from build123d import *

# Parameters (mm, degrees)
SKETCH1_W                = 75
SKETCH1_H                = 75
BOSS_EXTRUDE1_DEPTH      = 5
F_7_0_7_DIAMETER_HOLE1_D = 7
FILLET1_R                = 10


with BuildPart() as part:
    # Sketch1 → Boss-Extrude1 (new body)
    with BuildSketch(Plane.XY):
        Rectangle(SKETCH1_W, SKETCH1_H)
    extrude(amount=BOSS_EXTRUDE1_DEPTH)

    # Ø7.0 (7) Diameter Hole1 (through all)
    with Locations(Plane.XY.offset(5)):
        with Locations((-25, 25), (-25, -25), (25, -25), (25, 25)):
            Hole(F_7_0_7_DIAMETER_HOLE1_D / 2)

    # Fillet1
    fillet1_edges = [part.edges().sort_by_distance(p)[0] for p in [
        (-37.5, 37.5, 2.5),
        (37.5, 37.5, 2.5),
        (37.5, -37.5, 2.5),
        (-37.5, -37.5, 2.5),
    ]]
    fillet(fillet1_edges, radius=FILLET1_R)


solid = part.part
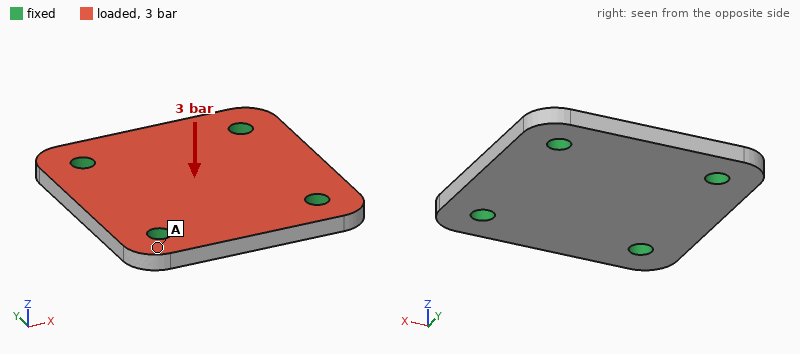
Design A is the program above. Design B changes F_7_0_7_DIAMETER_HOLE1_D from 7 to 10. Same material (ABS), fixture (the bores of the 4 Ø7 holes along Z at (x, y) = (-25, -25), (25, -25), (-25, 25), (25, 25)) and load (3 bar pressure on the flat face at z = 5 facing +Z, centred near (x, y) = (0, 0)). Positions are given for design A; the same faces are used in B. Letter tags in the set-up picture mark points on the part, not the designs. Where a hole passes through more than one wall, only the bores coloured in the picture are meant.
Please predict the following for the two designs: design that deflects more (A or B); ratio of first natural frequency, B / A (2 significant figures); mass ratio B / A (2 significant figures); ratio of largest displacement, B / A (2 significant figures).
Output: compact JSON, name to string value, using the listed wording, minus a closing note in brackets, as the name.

{"design that deflects more": "A", "ratio of first natural frequency, B / A": "1.1", "mass ratio B / A": "0.97", "ratio of largest displacement, B / A": "0.78"}
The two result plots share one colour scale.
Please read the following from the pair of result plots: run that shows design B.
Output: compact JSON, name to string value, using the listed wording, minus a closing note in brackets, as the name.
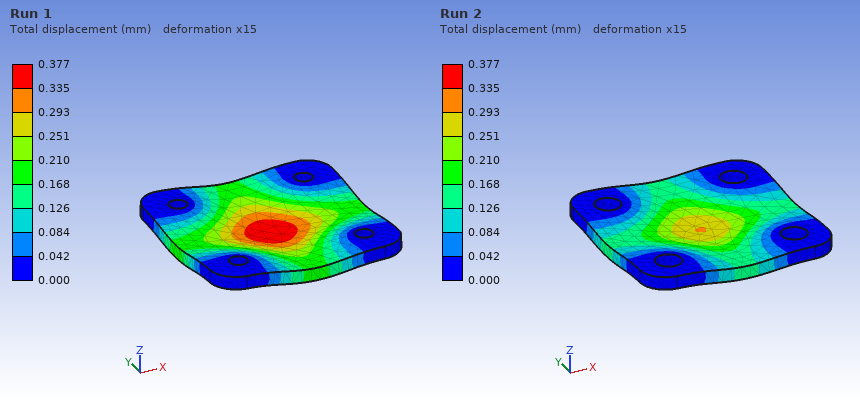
{"run that shows design B": "Run 2"}
